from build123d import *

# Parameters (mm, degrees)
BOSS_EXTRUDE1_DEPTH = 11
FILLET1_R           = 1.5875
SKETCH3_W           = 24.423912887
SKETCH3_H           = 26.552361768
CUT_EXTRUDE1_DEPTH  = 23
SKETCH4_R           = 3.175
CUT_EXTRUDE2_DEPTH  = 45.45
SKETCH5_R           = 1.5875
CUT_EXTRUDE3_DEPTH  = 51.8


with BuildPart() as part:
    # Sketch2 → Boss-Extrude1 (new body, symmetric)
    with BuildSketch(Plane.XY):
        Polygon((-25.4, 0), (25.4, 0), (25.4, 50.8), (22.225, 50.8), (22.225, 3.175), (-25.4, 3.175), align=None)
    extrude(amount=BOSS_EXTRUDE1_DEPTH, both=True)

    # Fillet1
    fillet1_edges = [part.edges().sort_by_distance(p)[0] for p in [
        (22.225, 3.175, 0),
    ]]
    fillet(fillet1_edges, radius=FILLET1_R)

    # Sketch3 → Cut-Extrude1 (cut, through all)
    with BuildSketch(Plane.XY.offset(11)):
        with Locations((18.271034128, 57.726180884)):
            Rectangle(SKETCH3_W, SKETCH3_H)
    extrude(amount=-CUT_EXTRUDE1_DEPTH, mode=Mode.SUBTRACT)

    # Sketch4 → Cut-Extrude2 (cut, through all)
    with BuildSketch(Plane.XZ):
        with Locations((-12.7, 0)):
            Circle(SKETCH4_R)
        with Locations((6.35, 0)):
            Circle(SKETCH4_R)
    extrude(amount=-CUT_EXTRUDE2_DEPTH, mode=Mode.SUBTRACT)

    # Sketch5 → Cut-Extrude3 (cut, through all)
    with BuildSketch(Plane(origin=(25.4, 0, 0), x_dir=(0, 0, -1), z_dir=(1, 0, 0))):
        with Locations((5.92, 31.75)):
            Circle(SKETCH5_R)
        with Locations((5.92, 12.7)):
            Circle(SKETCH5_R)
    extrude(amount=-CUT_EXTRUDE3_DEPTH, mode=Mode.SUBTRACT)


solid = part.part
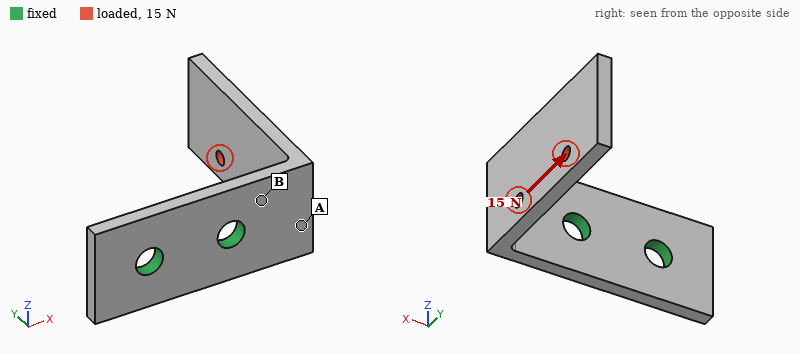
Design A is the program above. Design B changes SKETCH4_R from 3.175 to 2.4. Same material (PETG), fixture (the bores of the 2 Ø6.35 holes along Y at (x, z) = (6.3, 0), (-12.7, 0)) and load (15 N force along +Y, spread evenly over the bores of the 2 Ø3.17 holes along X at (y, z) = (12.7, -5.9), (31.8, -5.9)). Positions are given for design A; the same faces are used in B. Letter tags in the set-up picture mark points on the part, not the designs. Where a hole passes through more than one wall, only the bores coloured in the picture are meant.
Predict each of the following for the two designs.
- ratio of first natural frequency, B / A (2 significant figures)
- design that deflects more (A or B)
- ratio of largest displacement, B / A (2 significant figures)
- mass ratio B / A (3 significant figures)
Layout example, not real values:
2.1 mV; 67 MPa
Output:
0.97; B; 1.1; 1.01
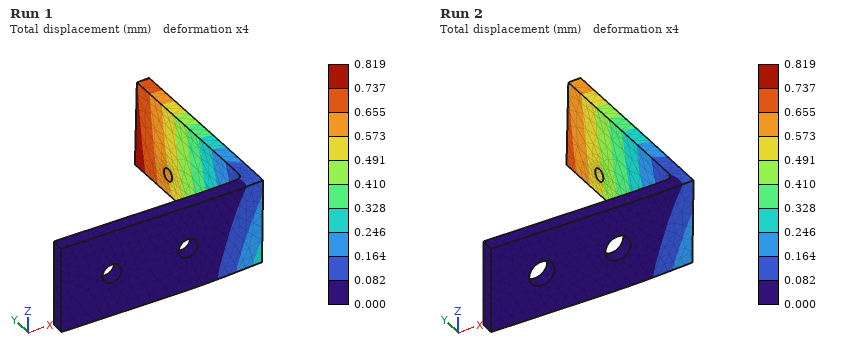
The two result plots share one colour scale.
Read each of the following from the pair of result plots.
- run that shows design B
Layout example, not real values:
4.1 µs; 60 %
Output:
Run 1
